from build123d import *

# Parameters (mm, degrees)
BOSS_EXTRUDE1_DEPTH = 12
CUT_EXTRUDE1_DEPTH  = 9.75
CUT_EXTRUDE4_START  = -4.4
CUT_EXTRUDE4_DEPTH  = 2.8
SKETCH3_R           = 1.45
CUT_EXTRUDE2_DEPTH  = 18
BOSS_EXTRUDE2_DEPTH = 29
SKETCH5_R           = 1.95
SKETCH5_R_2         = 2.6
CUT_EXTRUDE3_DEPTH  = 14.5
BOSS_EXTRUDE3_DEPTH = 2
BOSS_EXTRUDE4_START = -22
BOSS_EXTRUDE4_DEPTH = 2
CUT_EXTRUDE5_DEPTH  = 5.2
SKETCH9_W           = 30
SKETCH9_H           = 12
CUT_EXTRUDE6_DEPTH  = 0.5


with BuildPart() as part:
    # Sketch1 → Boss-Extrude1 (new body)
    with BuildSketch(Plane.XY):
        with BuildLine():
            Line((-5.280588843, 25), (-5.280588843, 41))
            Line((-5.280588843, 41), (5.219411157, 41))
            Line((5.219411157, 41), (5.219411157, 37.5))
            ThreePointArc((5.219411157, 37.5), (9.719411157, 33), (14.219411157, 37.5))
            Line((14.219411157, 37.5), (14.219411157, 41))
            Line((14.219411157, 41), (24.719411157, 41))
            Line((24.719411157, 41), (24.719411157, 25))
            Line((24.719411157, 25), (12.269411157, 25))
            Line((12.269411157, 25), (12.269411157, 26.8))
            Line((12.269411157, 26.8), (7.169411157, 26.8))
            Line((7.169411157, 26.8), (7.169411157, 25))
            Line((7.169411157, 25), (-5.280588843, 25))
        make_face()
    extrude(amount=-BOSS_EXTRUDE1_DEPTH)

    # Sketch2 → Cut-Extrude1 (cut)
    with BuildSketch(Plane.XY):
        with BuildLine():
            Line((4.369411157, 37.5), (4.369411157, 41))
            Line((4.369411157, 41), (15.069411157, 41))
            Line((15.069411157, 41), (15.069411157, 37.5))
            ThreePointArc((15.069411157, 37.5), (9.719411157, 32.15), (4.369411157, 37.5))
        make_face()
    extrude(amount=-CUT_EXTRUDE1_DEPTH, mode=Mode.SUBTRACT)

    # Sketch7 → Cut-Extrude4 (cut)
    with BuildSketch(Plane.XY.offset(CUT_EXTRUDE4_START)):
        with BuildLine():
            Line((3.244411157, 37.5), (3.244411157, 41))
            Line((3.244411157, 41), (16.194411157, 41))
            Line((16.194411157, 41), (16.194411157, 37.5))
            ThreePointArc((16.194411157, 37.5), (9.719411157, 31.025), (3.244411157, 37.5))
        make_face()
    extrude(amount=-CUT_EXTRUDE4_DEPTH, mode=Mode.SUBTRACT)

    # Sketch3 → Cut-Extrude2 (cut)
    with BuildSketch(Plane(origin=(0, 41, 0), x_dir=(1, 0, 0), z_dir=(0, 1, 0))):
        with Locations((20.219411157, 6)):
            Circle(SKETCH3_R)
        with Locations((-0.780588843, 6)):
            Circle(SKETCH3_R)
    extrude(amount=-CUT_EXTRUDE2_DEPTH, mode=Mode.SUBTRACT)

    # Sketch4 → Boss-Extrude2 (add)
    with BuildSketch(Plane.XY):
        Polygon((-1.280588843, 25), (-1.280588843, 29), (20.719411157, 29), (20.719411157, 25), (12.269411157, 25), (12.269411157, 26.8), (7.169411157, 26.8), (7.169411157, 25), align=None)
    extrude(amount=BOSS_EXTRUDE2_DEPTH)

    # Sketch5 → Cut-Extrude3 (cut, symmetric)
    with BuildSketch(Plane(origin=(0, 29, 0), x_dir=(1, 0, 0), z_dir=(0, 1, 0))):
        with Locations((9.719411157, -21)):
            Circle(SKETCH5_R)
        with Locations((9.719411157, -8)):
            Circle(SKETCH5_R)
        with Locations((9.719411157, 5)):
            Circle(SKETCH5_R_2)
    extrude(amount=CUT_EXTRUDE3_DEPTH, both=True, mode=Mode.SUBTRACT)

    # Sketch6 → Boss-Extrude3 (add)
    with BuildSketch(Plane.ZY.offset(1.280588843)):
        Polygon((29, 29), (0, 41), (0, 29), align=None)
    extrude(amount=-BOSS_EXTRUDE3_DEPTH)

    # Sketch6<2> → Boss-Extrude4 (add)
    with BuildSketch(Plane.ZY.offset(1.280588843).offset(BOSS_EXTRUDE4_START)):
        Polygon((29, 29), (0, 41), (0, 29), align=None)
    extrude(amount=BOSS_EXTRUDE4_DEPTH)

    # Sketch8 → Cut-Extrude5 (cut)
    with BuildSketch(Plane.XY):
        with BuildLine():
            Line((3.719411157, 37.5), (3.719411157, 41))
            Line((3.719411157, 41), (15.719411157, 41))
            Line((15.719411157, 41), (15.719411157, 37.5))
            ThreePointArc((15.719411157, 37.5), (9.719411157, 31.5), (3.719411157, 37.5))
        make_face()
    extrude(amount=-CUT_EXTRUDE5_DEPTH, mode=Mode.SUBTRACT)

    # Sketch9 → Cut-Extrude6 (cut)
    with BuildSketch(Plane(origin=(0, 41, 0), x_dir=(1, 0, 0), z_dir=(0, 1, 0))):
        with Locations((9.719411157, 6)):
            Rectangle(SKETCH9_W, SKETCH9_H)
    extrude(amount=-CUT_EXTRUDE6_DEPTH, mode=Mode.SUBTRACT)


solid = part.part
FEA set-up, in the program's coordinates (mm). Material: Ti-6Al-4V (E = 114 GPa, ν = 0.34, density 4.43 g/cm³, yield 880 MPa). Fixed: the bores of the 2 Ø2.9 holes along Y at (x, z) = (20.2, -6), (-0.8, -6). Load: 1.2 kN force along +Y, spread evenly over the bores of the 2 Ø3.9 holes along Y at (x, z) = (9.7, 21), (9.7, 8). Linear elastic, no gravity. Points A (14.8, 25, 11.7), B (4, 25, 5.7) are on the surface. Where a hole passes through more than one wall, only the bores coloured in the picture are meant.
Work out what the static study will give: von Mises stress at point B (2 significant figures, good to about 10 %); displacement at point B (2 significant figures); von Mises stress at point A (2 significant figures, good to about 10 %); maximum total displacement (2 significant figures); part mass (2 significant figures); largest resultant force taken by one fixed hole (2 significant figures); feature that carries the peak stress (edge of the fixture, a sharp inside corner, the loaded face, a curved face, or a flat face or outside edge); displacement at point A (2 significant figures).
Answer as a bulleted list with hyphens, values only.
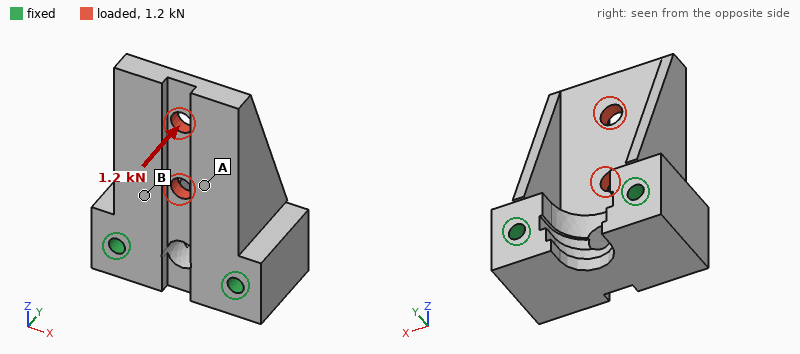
- 80 MPa
- 15 µm
- 38 MPa
- 79 µm
- 31 g
- 600 N
- the loaded face
- 29 µm
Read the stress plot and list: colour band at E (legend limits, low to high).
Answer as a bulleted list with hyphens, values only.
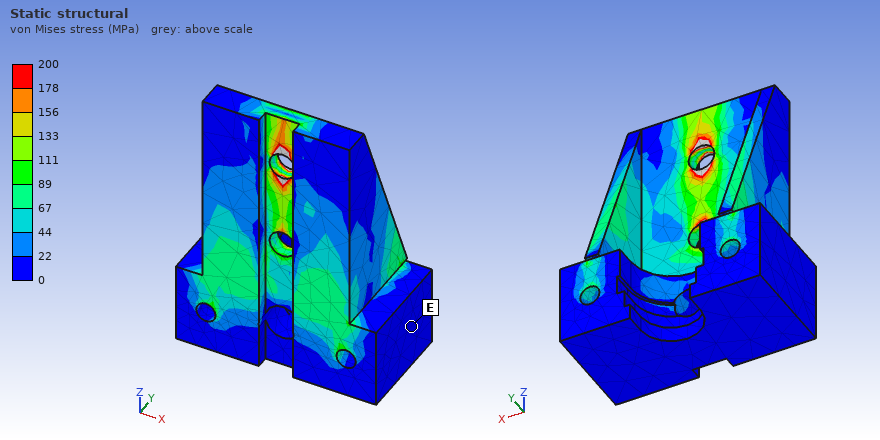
- 0 to 22 MPa
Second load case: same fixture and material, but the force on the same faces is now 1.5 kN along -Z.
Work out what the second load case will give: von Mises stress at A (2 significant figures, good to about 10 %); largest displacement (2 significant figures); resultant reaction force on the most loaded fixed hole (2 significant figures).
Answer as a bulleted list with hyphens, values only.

- 12 MPa
- 5.6 µm
- 770 N
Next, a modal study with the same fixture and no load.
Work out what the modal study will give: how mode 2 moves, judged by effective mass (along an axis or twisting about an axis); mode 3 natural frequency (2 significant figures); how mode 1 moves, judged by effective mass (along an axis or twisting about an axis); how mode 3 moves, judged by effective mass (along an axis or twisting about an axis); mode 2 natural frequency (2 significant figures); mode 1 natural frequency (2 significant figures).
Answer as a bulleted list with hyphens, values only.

- along X
- 17 kHz
- along Y
- along X
- 12 kHz
- 8700 Hz
